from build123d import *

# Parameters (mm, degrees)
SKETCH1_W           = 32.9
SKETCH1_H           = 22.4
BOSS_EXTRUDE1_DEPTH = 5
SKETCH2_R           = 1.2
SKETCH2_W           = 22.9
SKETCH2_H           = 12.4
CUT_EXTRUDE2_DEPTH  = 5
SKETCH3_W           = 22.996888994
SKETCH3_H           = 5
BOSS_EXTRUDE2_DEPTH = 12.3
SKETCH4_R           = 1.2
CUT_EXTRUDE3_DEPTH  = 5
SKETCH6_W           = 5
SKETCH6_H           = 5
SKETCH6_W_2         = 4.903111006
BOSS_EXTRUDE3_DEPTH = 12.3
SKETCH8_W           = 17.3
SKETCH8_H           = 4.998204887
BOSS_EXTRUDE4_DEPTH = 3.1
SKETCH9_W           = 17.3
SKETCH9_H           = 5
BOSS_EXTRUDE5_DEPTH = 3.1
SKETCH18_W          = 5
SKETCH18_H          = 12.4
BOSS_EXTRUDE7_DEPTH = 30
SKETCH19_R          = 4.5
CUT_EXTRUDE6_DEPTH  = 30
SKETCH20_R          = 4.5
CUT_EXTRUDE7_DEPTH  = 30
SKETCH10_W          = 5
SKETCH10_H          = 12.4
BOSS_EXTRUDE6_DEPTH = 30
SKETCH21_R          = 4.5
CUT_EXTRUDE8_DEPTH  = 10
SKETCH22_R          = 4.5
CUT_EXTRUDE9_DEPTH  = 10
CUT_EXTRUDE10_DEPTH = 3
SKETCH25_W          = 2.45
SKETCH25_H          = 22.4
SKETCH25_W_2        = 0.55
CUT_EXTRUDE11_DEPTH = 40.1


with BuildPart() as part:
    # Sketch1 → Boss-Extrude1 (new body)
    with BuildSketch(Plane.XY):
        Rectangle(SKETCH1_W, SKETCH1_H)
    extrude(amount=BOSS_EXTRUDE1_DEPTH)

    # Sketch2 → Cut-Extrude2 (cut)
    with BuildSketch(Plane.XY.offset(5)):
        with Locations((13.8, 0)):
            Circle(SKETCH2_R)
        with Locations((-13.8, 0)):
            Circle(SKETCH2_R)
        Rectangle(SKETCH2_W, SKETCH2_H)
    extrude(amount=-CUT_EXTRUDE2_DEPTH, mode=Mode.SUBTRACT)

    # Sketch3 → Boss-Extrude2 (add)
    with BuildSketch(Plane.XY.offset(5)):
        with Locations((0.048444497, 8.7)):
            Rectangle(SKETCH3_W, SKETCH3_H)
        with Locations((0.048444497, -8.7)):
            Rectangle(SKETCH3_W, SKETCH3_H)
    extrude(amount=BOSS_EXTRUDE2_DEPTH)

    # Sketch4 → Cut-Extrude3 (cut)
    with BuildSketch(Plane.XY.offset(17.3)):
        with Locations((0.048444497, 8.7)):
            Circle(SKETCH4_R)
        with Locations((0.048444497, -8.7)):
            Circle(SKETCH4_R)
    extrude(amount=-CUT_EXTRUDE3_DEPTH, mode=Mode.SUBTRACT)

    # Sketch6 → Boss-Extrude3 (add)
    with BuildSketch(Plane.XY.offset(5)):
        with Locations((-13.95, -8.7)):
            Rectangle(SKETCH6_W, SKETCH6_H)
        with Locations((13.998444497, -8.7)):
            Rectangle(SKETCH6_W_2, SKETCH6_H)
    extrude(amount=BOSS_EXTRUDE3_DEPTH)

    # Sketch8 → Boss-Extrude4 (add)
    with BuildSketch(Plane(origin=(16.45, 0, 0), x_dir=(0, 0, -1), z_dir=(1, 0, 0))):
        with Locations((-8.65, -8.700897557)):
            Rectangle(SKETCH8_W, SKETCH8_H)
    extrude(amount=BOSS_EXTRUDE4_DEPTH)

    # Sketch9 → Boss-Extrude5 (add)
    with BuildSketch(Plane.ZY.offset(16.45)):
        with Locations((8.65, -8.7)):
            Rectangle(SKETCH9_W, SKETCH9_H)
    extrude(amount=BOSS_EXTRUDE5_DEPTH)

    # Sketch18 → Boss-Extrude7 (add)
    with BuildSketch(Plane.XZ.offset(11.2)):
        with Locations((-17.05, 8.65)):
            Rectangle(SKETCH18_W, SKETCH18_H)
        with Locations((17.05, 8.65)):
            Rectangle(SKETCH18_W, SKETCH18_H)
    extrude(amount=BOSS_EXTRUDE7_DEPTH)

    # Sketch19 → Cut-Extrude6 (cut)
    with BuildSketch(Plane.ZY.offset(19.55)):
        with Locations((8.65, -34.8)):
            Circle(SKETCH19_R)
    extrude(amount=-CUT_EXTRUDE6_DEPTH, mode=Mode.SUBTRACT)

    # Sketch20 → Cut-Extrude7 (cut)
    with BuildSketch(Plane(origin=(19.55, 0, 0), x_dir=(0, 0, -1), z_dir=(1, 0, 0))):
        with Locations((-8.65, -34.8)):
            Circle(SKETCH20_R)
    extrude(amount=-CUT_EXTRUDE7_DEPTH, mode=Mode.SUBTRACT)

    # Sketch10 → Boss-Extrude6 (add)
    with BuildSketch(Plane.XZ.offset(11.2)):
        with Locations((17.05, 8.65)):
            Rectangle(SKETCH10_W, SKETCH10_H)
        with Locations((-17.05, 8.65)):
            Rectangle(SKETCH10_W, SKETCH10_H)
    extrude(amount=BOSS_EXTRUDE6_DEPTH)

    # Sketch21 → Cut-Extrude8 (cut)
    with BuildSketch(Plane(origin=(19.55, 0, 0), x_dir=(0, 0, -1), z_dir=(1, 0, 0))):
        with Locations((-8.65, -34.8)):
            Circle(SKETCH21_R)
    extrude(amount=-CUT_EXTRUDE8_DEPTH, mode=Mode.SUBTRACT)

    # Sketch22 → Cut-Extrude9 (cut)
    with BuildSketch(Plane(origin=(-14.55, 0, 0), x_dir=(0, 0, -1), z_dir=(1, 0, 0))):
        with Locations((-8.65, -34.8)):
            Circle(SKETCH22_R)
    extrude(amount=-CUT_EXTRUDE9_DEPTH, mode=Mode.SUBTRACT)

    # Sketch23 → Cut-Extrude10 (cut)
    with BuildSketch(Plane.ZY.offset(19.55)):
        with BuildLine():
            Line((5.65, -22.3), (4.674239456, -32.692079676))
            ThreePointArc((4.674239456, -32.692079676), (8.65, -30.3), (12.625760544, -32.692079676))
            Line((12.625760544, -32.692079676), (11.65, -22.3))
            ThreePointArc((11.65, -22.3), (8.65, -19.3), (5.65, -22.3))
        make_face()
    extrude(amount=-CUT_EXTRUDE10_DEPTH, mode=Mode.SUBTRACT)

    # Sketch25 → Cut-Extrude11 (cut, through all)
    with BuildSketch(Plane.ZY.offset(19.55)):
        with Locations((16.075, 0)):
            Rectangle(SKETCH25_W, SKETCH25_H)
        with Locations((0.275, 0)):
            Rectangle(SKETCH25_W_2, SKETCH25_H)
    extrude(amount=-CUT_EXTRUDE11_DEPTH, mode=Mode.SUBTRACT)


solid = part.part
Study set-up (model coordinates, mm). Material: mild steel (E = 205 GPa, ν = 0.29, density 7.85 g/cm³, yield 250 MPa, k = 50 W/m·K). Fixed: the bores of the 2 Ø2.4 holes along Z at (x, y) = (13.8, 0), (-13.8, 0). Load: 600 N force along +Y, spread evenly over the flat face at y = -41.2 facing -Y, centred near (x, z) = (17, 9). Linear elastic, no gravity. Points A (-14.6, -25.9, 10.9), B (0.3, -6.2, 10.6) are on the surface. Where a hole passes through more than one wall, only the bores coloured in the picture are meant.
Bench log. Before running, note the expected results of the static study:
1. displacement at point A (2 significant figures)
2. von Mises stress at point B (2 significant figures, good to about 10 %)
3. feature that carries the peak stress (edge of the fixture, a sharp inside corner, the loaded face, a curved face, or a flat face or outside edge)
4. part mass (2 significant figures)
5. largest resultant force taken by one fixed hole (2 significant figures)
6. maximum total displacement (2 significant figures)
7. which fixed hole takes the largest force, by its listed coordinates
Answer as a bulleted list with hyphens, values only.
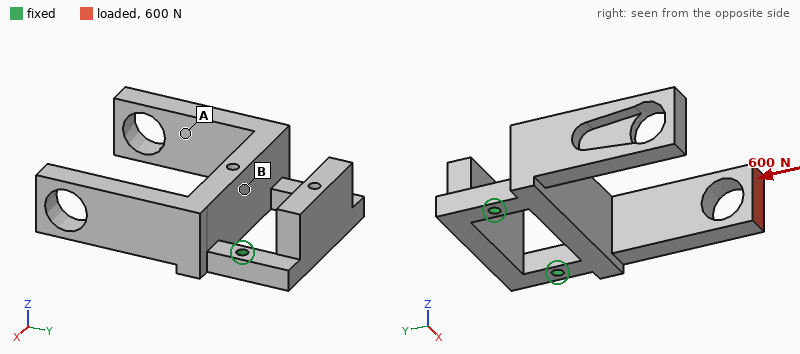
- 27 µm
- 27 MPa
- a flat face or outside edge
- 63 g
- 660 N
- 91 µm
- (13.8, 0)
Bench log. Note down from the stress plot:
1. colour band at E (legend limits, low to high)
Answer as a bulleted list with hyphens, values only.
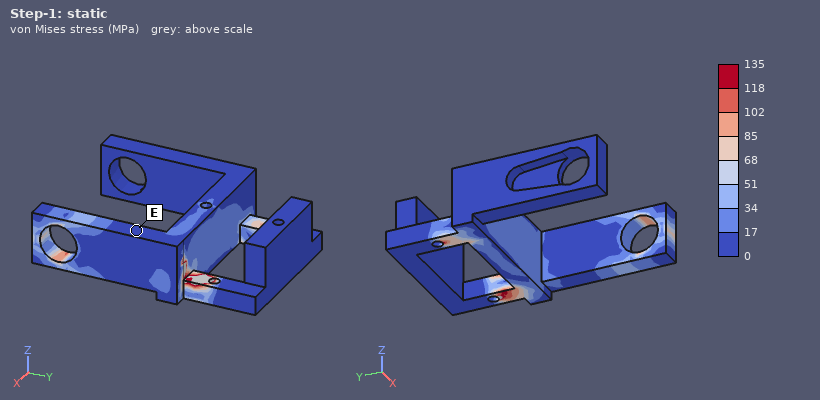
- 0 to 17 MPa
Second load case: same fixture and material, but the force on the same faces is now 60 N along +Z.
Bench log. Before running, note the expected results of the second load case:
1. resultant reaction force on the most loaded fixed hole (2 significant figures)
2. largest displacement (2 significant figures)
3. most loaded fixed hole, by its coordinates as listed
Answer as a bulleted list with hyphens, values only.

- 61 N
- 64 µm
- (13.8, 0)
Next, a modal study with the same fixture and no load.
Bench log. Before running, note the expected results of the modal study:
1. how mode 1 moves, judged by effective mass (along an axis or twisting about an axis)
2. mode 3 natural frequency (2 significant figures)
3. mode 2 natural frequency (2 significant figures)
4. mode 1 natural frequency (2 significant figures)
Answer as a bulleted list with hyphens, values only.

- along Z
- 3600 Hz
- 3200 Hz
- 1900 Hz
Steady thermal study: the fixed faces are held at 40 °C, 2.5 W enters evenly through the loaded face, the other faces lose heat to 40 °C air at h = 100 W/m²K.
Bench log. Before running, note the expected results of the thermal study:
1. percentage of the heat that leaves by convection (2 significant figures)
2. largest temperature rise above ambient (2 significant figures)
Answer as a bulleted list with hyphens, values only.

- 74 %
- 32 K
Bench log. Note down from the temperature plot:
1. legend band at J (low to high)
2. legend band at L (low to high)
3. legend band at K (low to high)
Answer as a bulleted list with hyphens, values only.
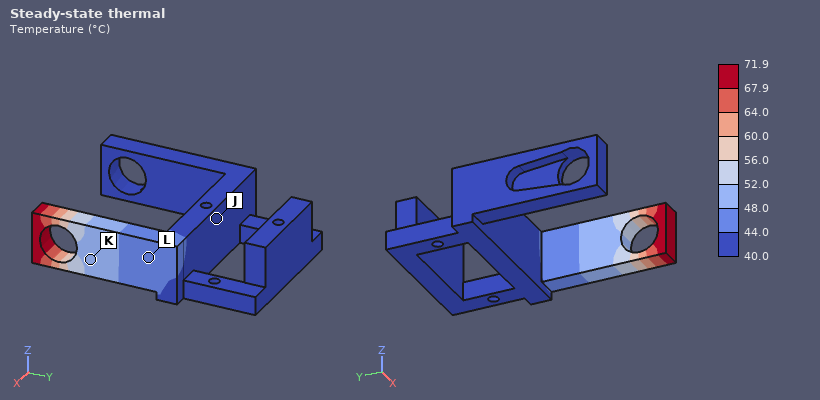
- 40.0 to 44.0 °C
- 44.0 to 48.0 °C
- 48.0 to 52.0 °C
